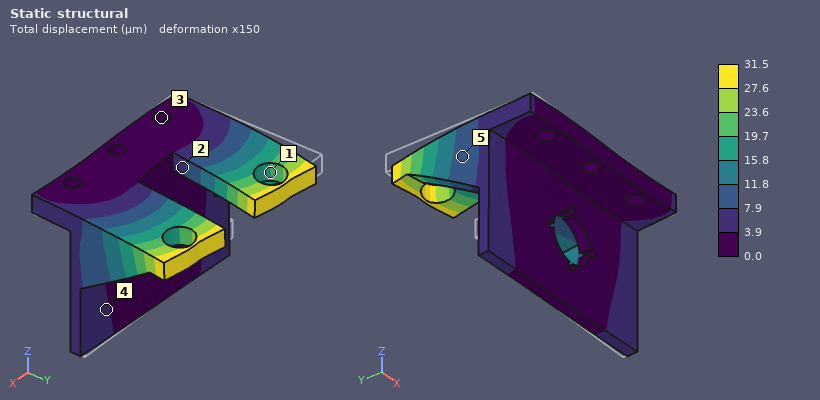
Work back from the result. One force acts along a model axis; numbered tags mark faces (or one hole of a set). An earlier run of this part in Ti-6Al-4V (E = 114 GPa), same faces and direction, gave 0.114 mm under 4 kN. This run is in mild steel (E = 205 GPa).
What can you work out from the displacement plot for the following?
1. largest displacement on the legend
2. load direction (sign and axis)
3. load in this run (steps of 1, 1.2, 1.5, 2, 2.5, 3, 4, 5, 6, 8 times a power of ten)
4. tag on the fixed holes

31.5 µm
+X
2 kN
3
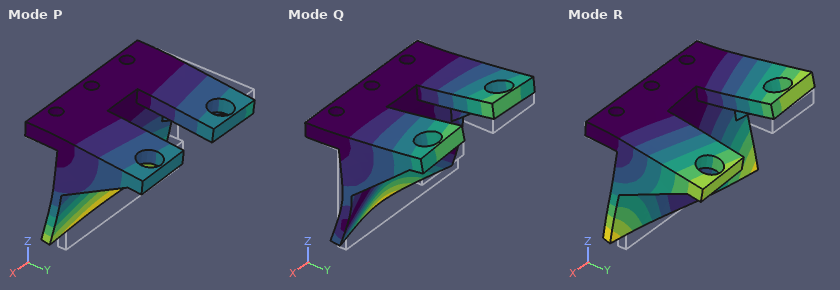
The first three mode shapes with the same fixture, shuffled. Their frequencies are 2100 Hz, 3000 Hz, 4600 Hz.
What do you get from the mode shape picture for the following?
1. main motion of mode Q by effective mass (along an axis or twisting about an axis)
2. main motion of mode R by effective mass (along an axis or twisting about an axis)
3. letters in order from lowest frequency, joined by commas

along Z
twisting about Y
P, R, Q
